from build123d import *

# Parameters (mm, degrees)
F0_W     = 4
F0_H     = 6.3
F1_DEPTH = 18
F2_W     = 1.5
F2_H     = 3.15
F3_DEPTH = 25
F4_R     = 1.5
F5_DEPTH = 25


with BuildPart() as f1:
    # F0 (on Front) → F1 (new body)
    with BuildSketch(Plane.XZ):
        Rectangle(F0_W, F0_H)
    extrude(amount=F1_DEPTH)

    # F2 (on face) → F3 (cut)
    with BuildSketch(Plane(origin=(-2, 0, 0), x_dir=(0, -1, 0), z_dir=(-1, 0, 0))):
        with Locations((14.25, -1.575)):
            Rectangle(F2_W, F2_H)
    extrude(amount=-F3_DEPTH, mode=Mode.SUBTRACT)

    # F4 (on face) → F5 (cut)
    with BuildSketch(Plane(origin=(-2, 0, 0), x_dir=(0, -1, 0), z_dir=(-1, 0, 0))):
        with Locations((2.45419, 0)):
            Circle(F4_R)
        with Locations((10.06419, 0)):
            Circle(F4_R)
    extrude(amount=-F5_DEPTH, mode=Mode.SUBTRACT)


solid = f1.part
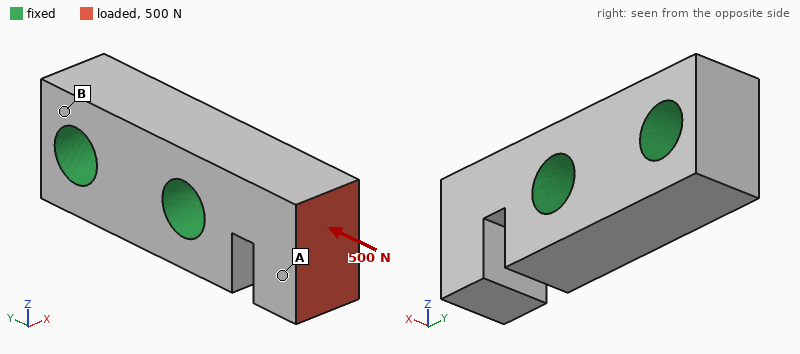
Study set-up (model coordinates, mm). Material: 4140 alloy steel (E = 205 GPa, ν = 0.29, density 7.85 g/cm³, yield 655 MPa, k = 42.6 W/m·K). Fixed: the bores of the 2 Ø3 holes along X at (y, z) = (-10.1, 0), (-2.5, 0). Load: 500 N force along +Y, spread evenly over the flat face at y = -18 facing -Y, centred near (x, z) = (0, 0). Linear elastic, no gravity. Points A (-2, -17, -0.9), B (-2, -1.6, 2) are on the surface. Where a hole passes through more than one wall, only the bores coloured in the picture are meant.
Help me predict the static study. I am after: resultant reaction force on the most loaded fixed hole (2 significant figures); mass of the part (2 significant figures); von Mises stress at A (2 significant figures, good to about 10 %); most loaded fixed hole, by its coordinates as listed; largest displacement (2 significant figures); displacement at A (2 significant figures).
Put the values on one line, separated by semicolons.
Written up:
490 N; 3.0 g; 45 MPa; (-10.1, 0); 10 µm; 6.1 µm
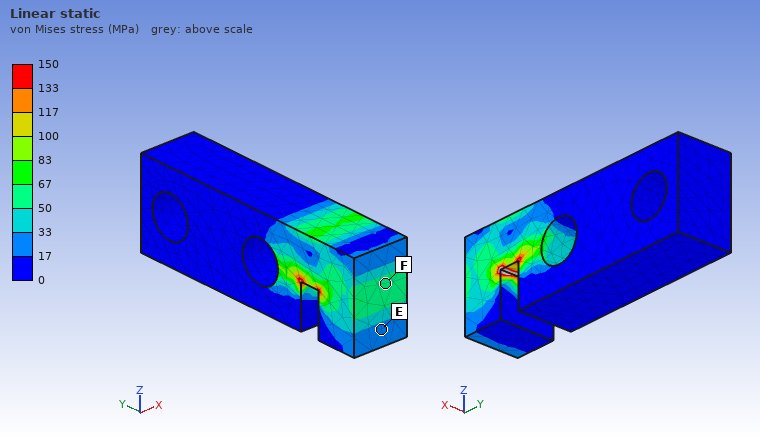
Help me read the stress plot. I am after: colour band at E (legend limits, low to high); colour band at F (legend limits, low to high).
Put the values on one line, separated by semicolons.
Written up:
17 to 33 MPa; 50 to 67 MPa
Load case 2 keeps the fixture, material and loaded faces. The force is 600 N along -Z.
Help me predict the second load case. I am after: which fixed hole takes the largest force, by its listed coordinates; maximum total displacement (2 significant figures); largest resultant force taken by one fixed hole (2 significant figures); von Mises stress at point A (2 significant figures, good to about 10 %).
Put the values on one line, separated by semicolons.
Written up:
(-10.1, 0); 36 µm; 730 N; 34 MPa
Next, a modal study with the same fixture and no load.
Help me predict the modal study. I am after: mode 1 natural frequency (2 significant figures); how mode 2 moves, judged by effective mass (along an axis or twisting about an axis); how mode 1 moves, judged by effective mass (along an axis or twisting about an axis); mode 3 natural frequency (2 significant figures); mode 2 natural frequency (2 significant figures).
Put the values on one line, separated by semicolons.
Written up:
37 kHz; along X; along Z; 68 kHz; 39 kHz
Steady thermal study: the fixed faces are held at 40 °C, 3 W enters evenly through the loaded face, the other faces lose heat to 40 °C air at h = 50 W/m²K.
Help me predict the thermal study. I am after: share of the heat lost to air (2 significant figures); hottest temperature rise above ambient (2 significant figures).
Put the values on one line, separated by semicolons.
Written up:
4.3 %; 34 K
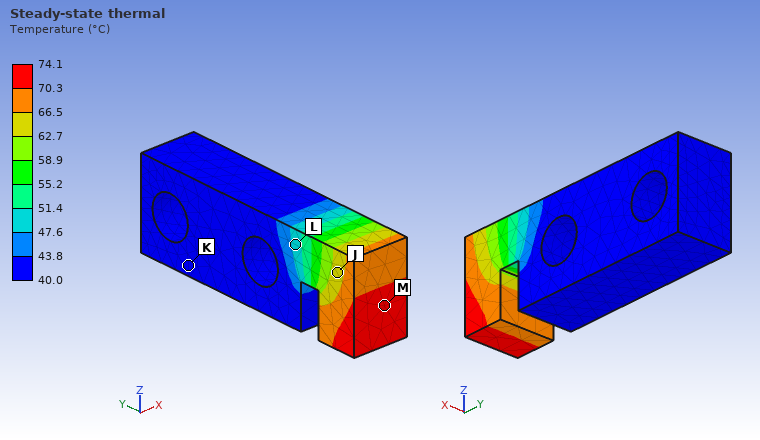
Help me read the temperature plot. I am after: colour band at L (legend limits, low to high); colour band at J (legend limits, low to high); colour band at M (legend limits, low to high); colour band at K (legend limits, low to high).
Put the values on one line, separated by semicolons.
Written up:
47.6 to 51.4 °C; 62.7 to 66.5 °C; 70.3 to 74.1 °C; 40.0 to 43.8 °C
